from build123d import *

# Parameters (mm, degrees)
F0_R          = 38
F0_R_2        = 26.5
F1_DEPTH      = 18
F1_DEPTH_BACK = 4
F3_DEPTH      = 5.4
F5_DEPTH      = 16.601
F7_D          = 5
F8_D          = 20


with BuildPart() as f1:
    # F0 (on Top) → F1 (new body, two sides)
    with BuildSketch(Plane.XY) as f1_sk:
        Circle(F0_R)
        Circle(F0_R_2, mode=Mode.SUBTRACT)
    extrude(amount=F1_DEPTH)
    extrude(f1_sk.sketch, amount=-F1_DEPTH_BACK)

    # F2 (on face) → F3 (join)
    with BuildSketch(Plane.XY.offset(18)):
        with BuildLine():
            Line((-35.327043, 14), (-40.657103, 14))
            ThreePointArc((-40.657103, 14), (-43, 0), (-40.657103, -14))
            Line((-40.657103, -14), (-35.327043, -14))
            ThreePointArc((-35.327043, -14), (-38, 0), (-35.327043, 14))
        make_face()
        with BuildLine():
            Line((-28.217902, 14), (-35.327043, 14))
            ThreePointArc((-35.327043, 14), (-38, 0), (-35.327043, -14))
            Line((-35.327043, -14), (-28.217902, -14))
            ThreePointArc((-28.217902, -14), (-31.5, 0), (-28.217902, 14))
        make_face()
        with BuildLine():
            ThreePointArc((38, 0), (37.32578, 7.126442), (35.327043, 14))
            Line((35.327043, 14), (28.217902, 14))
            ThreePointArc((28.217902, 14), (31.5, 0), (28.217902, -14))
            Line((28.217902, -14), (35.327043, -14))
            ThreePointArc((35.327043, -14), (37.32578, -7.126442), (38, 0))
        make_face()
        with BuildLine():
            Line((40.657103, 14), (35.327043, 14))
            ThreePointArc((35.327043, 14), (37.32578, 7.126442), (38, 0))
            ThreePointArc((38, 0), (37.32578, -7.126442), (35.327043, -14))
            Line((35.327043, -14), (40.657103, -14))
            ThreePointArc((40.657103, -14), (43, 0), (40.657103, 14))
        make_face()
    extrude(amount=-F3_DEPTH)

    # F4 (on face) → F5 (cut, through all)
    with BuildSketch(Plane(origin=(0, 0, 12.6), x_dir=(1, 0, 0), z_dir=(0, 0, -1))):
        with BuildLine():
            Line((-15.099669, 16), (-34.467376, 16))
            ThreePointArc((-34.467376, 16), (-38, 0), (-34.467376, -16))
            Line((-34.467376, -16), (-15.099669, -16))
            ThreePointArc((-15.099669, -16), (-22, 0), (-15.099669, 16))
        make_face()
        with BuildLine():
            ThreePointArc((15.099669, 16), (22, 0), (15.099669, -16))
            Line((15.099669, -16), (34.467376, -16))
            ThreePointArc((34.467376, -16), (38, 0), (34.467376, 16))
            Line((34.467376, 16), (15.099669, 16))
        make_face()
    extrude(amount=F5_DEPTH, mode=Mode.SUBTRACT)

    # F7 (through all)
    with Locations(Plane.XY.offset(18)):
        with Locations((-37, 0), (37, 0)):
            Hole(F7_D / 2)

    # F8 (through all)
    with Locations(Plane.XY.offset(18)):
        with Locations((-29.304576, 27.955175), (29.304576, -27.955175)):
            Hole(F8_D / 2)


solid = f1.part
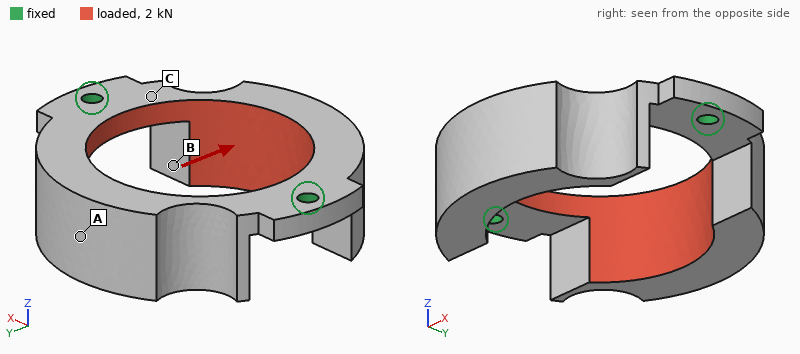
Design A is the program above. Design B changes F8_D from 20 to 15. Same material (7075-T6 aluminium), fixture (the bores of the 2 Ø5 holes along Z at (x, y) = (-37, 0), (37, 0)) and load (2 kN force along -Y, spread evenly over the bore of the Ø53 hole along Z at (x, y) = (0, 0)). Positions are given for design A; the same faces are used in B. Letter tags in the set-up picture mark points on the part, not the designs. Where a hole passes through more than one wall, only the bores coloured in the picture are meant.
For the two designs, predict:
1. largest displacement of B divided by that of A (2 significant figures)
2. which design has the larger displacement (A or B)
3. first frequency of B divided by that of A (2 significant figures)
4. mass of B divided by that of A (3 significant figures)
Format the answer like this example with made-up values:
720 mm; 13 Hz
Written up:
0.88; A; 1.0; 1.06
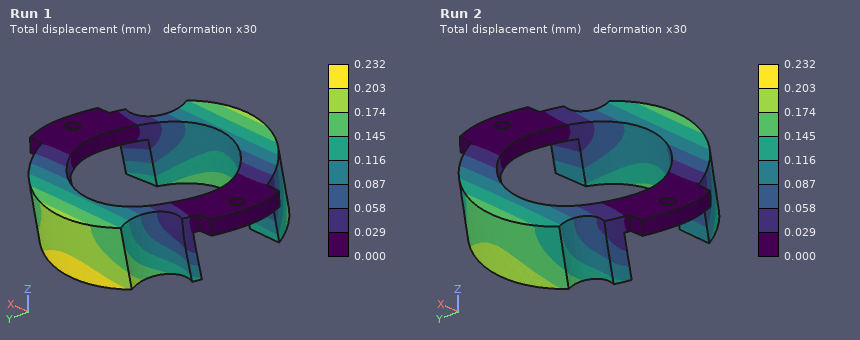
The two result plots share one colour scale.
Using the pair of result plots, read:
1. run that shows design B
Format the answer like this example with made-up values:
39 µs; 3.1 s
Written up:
Run 2
